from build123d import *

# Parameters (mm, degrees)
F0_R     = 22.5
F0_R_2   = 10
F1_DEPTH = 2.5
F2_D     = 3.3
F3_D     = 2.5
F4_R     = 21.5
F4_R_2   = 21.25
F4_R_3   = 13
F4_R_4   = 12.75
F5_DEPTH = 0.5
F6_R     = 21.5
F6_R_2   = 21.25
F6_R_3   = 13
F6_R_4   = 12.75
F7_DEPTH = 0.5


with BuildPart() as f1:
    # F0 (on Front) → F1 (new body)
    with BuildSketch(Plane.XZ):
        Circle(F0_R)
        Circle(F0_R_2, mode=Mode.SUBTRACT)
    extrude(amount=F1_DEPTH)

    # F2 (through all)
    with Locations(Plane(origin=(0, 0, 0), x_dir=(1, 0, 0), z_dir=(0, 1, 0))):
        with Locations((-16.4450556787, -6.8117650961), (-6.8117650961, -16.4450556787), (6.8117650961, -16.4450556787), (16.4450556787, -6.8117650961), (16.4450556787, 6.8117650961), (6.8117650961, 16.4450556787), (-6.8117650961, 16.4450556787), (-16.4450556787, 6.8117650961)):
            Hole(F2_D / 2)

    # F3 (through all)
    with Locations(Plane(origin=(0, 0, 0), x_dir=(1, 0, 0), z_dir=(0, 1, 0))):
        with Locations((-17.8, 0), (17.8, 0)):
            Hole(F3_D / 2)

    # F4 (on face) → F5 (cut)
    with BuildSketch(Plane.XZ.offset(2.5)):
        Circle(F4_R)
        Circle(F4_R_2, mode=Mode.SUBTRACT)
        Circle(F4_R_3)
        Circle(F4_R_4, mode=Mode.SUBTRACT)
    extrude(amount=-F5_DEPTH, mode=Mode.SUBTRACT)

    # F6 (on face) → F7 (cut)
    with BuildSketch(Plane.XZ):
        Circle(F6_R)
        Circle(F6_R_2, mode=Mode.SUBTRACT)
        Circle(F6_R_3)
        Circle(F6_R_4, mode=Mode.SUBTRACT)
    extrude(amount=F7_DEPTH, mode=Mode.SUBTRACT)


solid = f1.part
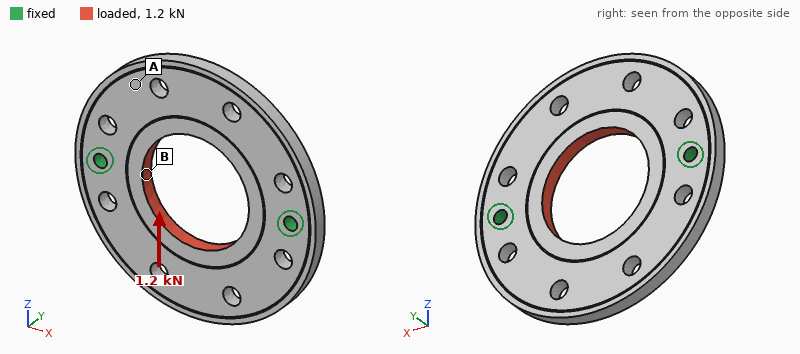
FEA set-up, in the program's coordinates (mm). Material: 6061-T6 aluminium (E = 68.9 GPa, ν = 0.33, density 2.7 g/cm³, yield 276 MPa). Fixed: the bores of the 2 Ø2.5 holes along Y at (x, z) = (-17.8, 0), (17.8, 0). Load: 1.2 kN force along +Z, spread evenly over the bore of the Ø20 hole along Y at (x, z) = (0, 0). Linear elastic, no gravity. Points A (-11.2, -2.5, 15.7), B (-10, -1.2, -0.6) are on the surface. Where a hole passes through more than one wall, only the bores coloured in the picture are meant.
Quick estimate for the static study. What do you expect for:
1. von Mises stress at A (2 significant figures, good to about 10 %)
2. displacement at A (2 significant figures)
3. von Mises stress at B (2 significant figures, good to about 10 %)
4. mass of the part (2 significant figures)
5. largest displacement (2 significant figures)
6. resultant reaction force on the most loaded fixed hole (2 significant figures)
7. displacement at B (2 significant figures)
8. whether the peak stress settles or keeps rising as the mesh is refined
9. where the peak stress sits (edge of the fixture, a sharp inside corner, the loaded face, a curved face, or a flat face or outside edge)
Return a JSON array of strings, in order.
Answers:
["7.2 MPa", "4.5 µm", "13 MPa", "7.9 g", "6.8 µm", "600 N", "4.7 µm", "keeps rising", "edge of the fixture"]
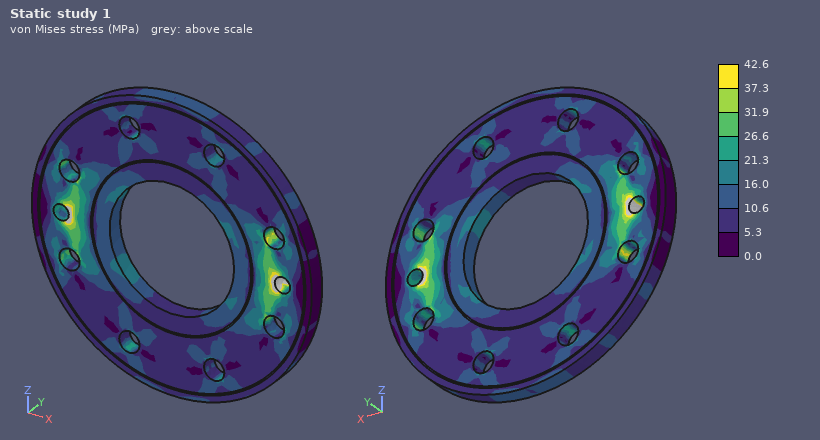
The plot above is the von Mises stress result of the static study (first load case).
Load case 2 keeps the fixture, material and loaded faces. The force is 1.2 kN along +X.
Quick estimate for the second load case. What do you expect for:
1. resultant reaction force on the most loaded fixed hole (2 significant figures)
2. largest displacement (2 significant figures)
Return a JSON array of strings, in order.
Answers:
["600 N", "7.0 µm"]
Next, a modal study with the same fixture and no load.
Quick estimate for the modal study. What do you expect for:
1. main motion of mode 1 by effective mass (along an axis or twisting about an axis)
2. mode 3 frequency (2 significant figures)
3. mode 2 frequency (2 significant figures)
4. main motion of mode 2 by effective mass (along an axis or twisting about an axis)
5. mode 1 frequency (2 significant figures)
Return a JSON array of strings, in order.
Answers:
["twisting about X", "9000 Hz", "3700 Hz", "along Y", "3300 Hz"]
